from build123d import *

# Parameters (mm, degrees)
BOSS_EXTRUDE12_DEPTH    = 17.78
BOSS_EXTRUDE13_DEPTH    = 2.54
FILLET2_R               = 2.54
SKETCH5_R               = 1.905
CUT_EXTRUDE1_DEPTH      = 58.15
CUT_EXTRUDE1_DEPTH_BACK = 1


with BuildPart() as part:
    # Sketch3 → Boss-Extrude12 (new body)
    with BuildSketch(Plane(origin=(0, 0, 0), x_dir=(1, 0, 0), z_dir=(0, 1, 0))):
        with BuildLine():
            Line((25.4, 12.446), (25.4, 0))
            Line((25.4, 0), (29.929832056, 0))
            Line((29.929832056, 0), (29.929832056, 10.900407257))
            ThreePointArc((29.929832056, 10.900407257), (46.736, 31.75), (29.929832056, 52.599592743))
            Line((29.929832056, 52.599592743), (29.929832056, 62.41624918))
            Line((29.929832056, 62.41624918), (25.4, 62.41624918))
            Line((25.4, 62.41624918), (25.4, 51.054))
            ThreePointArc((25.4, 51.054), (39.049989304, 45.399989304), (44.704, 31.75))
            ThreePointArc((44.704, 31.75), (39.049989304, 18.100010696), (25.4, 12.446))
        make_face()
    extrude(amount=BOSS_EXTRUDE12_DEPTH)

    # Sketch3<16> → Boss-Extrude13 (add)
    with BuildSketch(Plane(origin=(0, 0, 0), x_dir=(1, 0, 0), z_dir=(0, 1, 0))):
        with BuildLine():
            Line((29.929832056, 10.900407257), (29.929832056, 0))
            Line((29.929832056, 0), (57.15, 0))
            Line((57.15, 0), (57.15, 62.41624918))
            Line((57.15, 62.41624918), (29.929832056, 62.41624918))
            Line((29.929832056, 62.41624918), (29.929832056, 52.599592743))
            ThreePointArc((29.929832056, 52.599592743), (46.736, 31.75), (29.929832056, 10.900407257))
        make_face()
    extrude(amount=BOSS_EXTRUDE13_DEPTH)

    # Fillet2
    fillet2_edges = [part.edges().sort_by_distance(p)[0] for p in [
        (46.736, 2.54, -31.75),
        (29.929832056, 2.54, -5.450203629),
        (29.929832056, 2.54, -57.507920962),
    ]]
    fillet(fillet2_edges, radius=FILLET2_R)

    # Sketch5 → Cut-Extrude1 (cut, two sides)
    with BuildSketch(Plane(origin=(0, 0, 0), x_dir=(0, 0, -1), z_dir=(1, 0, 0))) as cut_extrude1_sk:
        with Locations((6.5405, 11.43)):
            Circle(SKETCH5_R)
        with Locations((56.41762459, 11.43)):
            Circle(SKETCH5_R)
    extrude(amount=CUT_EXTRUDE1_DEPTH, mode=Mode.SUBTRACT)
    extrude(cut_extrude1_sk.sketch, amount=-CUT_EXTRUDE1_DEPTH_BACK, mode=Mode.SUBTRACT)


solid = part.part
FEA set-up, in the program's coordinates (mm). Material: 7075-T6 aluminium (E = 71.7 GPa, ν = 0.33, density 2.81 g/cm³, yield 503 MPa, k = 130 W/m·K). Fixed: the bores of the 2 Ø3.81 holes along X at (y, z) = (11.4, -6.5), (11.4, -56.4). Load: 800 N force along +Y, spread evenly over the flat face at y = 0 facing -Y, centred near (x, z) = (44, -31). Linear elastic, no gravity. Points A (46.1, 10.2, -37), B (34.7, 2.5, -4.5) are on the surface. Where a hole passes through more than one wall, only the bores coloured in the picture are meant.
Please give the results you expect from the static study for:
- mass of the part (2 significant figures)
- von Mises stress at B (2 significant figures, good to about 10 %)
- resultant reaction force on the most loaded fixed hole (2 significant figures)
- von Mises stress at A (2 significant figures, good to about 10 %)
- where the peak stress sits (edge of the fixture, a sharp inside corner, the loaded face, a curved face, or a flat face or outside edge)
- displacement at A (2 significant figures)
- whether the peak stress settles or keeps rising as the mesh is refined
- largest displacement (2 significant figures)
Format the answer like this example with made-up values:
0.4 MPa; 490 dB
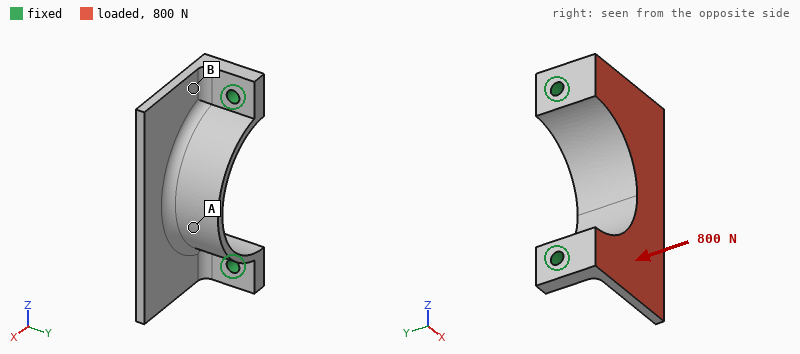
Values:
19 g; 41 MPa; 410 N; 17 MPa; edge of the fixture; 0.064 mm; keeps rising; 0.23 mm
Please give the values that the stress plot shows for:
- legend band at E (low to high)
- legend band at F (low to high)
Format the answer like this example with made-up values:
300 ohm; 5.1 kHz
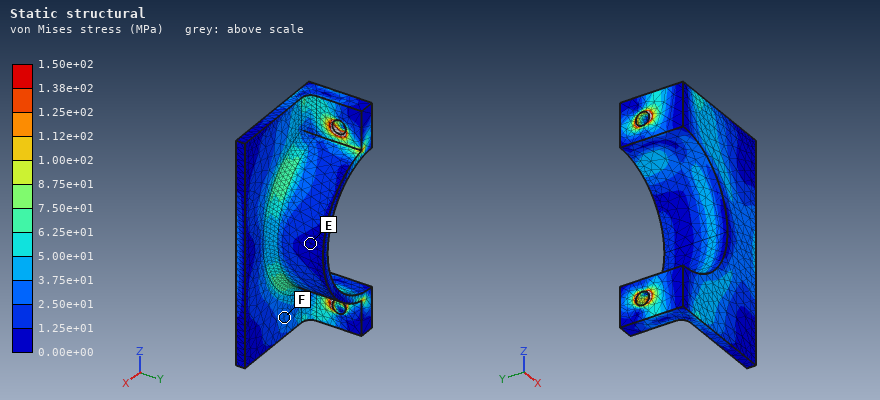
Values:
0.00e+00 to 1.25e+01 MPa; 2.50e+01 to 3.75e+01 MPa
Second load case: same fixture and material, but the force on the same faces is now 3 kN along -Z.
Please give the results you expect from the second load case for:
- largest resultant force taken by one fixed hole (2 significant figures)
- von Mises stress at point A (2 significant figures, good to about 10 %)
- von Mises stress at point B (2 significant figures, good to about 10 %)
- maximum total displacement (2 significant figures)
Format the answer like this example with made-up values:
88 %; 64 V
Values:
1.8 kN; 32 MPa; 31 MPa; 86 µm
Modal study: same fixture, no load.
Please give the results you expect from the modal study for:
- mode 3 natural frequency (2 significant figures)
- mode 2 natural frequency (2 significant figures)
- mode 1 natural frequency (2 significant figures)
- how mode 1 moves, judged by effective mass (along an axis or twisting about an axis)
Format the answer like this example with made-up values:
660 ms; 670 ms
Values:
7600 Hz; 4500 Hz; 3800 Hz; along Y
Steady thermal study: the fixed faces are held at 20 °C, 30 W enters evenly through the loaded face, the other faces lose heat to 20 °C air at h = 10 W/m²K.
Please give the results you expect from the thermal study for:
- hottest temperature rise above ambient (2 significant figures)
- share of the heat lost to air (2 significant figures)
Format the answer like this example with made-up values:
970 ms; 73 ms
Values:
37 K; 3.2 %
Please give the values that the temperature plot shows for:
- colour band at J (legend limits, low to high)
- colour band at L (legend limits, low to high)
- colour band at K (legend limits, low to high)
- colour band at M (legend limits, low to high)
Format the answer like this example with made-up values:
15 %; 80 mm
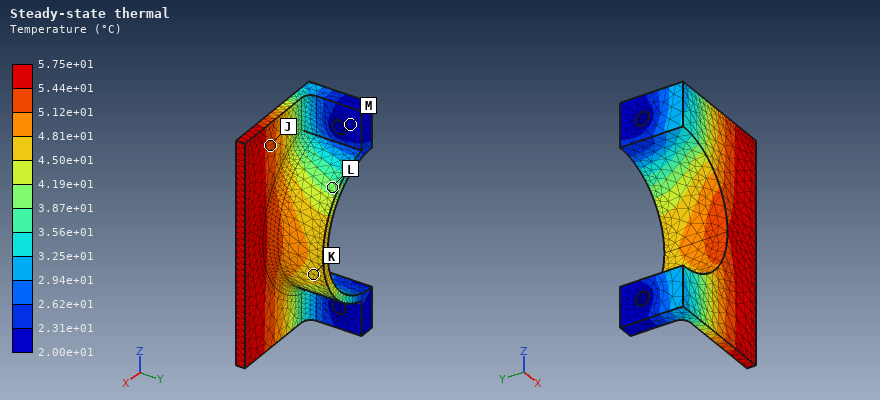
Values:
5.12e+01 to 5.44e+01 °C; 3.87e+01 to 4.19e+01 °C; 4.50e+01 to 4.81e+01 °C; 2.00e+01 to 2.31e+01 °C
